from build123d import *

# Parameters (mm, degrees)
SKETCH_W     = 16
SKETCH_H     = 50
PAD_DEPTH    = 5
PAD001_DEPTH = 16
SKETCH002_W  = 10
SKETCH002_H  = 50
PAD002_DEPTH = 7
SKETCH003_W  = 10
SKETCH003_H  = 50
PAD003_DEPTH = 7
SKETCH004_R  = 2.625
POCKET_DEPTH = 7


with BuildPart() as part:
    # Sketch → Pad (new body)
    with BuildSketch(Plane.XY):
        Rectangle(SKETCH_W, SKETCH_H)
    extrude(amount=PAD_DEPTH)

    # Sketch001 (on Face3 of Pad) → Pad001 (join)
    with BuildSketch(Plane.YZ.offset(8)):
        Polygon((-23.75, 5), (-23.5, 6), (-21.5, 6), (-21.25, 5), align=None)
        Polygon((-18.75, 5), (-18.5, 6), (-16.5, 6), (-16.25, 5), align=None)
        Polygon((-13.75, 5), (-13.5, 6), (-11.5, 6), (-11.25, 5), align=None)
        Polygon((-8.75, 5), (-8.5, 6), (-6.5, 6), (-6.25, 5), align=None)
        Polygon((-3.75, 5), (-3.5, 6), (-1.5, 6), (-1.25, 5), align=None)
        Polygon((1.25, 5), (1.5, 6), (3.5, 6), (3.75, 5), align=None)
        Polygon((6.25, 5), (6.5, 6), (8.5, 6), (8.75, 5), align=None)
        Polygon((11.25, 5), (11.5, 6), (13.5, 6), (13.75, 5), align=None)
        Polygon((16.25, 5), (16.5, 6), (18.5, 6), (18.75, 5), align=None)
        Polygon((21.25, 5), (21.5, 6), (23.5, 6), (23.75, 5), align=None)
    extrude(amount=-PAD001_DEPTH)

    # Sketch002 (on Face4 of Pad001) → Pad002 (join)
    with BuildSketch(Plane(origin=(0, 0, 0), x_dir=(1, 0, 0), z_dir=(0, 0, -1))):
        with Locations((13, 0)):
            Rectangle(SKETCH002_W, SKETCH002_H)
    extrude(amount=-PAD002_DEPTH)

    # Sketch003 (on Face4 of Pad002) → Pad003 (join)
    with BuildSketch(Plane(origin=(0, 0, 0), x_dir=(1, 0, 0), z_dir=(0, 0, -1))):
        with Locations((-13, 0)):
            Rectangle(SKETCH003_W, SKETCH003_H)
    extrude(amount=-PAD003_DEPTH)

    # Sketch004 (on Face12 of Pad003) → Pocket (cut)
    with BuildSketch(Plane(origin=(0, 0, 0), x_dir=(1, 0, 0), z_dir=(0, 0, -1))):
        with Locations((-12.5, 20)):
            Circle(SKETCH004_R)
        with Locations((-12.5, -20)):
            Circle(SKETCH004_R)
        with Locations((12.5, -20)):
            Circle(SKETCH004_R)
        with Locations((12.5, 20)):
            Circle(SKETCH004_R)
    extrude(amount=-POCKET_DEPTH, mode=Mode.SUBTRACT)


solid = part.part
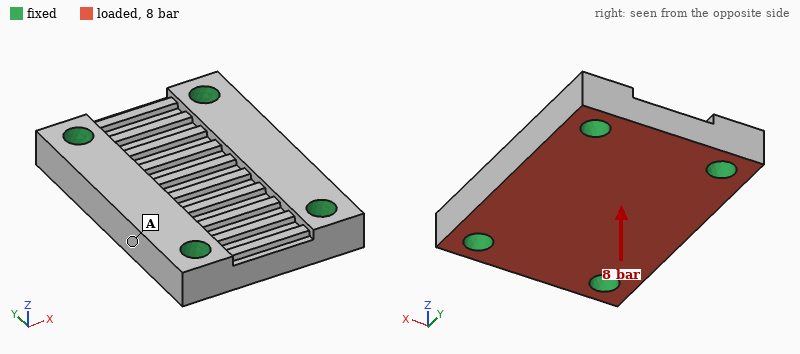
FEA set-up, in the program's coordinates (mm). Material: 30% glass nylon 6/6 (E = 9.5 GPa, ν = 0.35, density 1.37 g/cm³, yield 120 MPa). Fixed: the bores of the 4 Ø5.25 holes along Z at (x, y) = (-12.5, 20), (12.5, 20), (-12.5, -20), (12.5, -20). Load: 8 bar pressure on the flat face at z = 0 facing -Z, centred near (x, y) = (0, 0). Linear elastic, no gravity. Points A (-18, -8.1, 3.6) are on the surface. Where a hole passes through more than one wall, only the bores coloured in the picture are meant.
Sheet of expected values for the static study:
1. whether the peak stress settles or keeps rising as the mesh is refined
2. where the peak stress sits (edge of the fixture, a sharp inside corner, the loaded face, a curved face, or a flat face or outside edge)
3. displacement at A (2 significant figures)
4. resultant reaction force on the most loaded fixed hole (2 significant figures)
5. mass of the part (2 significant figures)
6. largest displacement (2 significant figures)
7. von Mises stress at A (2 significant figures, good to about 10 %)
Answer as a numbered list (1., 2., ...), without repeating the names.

1. keeps rising
2. edge of the fixture
3. 17 µm
4. 350 N
5. 15 g
6. 35 µm
7. 3.8 MPa
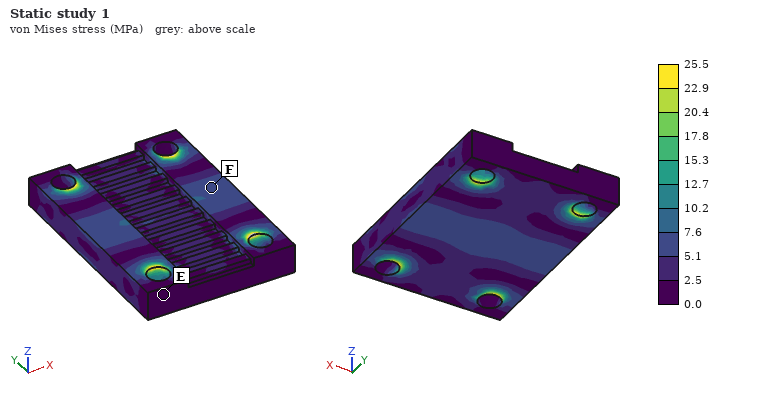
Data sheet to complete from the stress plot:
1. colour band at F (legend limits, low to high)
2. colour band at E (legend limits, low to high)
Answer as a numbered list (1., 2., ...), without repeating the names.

1. 5.1 to 7.6 MPa
2. 0.0 to 2.5 MPa
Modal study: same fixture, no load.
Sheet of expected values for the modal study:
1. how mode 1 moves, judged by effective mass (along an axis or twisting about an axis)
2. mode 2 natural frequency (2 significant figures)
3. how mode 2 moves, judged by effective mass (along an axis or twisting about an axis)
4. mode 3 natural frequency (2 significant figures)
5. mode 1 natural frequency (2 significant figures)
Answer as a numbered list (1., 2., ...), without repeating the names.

1. along Z
2. 13 kHz
3. twisting about Y
4. 17 kHz
5. 9900 Hz
